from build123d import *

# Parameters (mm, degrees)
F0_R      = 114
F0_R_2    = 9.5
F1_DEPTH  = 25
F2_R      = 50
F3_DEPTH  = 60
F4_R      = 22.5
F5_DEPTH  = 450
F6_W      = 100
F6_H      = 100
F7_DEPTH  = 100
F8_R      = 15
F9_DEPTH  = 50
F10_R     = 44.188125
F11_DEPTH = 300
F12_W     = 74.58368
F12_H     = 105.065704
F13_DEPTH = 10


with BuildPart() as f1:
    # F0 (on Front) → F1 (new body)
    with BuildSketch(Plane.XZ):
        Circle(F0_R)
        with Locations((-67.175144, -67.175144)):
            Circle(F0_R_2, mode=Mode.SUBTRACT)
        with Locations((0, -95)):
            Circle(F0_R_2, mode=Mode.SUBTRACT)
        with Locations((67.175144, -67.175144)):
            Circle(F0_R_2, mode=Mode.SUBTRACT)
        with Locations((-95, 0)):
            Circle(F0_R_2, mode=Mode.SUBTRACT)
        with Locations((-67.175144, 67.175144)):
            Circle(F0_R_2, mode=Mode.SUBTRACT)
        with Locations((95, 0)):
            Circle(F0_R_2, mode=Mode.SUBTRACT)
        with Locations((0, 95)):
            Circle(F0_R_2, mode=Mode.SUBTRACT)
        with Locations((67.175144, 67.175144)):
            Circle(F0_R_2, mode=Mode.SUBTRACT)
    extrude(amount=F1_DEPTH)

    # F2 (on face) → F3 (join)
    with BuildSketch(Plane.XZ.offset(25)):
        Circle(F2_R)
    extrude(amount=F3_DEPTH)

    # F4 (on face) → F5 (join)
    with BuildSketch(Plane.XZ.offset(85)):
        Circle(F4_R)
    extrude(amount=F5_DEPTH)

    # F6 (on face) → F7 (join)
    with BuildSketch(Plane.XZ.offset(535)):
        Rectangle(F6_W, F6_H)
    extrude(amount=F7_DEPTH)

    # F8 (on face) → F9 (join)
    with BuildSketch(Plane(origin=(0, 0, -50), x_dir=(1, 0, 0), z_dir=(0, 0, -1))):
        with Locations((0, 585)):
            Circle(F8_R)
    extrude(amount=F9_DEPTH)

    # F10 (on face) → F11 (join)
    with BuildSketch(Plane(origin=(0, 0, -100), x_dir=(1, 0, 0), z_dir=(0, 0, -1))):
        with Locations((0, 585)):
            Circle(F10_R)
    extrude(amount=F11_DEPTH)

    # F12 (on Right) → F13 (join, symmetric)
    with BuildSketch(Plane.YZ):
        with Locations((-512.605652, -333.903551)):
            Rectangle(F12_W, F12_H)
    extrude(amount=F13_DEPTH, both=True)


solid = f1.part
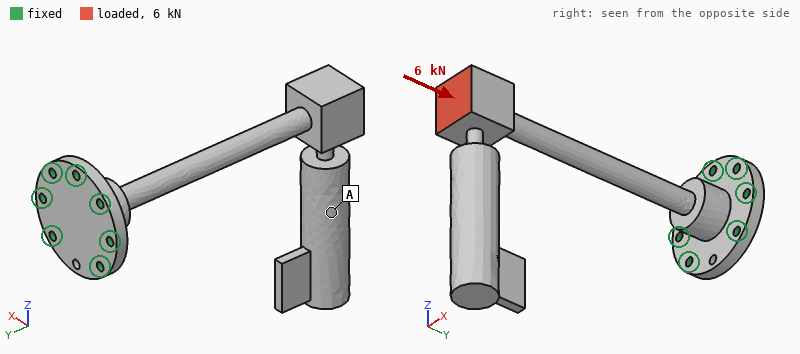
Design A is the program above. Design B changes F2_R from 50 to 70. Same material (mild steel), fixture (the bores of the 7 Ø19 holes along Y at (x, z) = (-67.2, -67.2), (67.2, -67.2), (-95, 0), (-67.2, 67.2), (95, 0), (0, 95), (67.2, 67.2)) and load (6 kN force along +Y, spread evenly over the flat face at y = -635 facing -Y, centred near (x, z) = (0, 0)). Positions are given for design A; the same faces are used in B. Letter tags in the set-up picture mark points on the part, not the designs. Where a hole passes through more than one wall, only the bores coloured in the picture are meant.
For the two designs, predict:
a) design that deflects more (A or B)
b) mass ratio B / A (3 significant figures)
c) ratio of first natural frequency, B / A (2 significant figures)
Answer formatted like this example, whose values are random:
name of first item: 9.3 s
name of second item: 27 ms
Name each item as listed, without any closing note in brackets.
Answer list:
design that deflects more: A
mass ratio B / A: 1.09
ratio of first natural frequency, B / A: 1.0
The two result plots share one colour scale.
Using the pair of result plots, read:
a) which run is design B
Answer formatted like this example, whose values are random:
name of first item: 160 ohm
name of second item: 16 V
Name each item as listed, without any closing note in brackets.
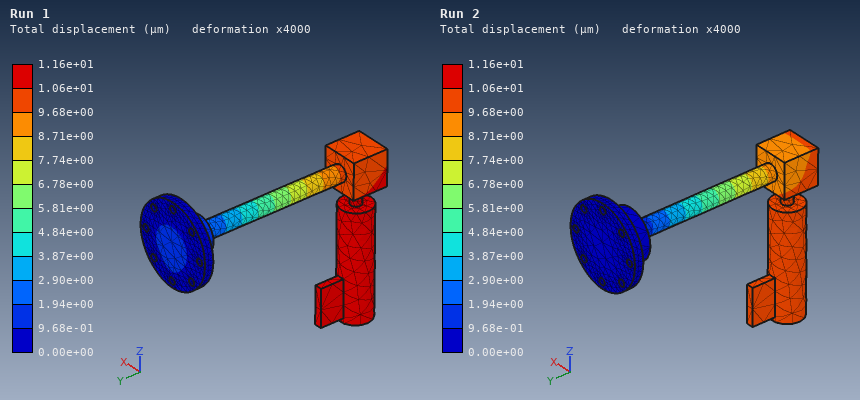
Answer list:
which run is design B: Run 2
